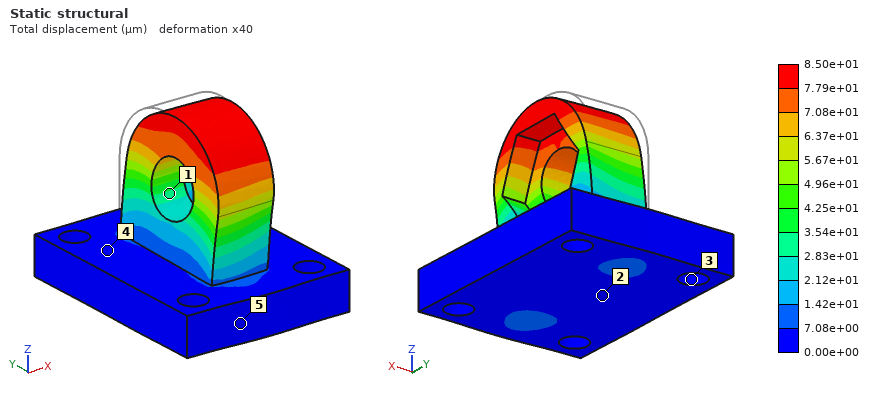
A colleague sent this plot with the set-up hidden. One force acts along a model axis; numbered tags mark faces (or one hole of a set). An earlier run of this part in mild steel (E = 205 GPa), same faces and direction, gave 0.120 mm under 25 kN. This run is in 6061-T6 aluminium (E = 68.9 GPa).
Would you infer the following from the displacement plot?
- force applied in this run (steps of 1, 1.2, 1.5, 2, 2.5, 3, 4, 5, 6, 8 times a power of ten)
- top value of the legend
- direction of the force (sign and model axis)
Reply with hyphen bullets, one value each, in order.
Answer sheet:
- 6 kN
- 8.50e+01 µm
- -Y
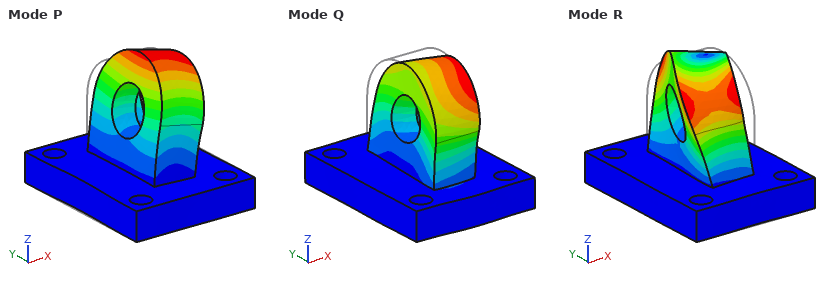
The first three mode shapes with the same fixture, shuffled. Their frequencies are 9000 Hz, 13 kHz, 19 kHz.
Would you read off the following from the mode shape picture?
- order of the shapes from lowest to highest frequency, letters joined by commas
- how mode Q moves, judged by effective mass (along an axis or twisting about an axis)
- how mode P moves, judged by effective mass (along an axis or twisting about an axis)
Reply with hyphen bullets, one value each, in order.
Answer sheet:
- P, Q, R
- along Y
- along X
